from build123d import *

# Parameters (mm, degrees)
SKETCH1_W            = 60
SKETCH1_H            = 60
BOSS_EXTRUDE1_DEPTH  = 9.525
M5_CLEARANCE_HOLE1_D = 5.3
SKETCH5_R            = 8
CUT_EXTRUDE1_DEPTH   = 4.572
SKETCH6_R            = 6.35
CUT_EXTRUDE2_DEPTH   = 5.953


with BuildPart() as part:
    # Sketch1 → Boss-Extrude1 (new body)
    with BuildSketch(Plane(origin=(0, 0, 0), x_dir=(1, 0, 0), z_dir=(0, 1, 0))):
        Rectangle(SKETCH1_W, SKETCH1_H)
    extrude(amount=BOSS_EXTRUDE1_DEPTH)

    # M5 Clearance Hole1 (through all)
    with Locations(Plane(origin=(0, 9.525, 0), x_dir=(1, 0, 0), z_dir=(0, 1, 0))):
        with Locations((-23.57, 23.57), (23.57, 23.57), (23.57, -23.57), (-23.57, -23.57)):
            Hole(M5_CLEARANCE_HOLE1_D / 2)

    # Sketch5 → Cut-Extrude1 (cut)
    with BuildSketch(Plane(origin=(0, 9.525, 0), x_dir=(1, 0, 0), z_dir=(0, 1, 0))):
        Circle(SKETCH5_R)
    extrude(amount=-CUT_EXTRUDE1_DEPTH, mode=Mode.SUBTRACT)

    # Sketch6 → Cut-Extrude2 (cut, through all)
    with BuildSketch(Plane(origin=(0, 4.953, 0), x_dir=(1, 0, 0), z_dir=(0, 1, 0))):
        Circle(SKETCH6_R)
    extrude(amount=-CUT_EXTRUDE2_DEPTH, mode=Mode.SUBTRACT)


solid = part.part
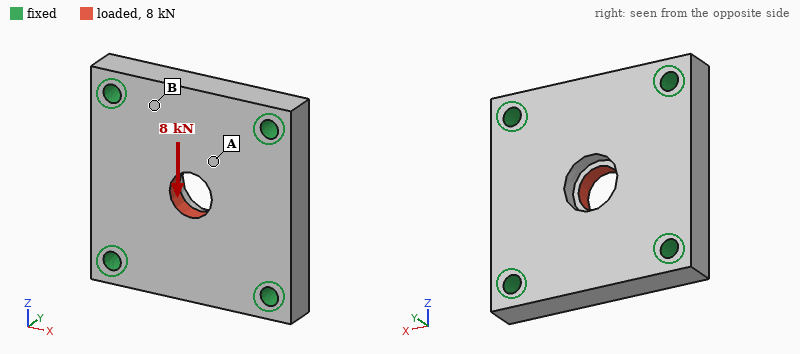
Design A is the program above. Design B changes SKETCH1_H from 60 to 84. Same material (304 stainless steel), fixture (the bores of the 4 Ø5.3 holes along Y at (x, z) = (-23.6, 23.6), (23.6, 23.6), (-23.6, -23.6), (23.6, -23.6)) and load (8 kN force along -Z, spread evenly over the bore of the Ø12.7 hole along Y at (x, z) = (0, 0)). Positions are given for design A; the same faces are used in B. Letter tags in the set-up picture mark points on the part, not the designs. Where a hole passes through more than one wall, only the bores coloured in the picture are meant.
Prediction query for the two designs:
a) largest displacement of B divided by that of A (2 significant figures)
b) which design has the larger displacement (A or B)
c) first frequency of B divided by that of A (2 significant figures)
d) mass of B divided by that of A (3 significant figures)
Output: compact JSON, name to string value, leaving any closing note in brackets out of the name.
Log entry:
{"largest displacement of B divided by that of A": "0.89", "which design has the larger displacement": "A", "first frequency of B divided by that of A": "1.0", "mass of B divided by that of A": "1.43"}
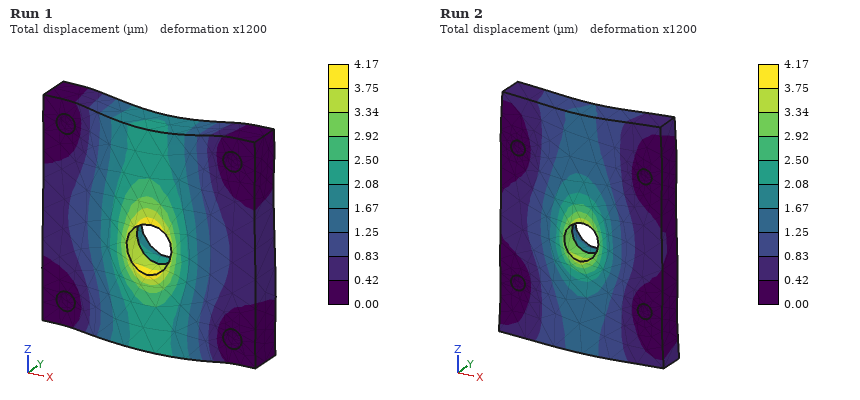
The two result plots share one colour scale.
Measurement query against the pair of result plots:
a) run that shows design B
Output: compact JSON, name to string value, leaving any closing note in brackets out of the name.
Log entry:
{"run that shows design B": "Run 2"}
